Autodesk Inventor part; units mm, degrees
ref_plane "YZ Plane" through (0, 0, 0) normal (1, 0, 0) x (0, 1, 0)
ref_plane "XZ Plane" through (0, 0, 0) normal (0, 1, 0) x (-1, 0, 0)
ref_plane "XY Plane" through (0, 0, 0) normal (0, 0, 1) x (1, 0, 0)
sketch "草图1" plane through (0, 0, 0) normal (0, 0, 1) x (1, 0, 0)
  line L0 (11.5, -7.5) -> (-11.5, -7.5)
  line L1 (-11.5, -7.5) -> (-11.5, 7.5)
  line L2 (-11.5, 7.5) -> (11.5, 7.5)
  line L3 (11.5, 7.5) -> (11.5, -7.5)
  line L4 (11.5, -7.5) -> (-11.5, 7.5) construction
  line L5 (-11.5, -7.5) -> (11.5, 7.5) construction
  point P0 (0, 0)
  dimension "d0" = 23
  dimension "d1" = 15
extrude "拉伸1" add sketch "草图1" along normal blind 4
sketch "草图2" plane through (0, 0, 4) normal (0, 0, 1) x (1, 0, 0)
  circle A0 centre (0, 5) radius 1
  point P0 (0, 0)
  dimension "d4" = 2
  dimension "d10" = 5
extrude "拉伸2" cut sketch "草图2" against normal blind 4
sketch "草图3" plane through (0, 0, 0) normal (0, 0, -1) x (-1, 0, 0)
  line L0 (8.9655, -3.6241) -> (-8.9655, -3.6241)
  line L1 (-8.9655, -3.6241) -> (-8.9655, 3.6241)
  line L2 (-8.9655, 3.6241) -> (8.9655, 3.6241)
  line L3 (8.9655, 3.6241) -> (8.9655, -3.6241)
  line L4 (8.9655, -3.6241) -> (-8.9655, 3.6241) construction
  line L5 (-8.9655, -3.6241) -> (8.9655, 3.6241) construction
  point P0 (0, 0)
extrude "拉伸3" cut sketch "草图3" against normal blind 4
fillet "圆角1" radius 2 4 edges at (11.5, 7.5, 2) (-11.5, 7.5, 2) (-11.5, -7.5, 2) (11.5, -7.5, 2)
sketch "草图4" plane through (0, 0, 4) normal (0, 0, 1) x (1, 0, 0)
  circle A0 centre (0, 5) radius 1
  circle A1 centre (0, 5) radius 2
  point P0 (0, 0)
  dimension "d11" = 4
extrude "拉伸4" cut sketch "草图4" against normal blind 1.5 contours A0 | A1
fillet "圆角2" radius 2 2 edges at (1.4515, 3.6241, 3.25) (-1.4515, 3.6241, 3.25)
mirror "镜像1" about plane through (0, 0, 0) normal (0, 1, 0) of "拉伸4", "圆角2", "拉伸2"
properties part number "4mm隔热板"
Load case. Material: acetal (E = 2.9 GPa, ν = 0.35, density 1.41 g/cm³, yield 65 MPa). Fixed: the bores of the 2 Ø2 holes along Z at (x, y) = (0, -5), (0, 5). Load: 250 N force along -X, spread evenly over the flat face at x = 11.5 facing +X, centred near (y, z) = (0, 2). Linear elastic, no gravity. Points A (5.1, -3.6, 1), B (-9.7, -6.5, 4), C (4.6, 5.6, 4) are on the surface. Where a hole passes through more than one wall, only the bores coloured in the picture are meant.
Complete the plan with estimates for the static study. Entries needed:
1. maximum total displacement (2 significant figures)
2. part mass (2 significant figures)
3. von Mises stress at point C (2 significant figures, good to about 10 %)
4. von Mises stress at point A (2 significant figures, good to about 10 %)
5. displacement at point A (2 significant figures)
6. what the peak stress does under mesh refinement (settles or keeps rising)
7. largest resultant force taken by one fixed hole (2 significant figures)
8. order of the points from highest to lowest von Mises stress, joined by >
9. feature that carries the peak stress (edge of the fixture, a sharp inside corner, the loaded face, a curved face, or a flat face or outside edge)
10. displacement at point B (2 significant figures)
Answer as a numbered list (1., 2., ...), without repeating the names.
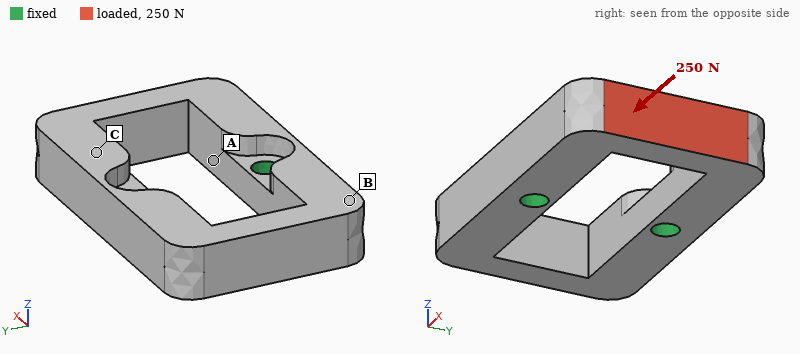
1. 0.17 mm
2. 1.1 g
3. 11 MPa
4. 18 MPa
5. 0.041 mm
6. keeps rising
7. 130 N
8. A > C > B
9. edge of the fixture
10. 0.027 mm
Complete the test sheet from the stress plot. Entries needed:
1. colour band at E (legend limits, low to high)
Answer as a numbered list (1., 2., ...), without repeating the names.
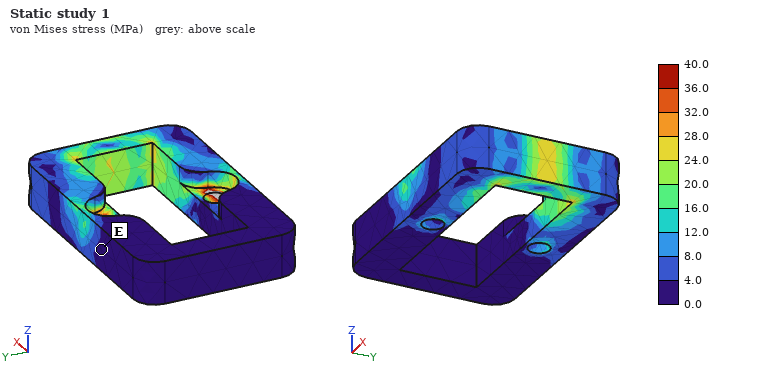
1. 0.0 to 4.0 MPa
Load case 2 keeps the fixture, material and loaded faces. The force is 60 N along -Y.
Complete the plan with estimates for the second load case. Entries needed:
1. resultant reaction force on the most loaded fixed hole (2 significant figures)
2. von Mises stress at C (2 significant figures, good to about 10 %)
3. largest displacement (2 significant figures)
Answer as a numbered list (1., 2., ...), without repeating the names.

1. 44 N
2. 4.9 MPa
3. 0.15 mm
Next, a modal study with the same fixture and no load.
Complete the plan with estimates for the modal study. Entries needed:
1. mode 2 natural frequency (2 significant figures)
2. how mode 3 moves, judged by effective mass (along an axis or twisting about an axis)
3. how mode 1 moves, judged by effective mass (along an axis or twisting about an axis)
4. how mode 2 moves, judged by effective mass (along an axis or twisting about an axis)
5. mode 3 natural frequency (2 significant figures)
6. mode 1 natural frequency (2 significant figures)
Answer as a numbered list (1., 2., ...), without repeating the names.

1. 4200 Hz
2. twisting about Z
3. twisting about Y
4. along Z
5. 5600 Hz
6. 3600 Hz
